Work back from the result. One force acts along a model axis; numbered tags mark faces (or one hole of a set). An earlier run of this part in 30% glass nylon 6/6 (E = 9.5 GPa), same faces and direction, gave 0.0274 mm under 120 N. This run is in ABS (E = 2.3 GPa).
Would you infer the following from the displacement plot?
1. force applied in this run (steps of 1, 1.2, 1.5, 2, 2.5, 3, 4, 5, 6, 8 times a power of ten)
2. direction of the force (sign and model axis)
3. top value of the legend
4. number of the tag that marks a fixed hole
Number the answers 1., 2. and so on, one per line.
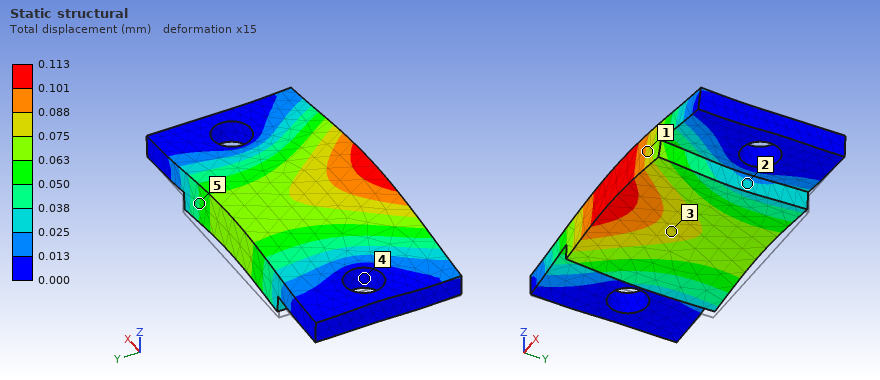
1. 120 N
2. +Z
3. 0.113 mm
4. 4
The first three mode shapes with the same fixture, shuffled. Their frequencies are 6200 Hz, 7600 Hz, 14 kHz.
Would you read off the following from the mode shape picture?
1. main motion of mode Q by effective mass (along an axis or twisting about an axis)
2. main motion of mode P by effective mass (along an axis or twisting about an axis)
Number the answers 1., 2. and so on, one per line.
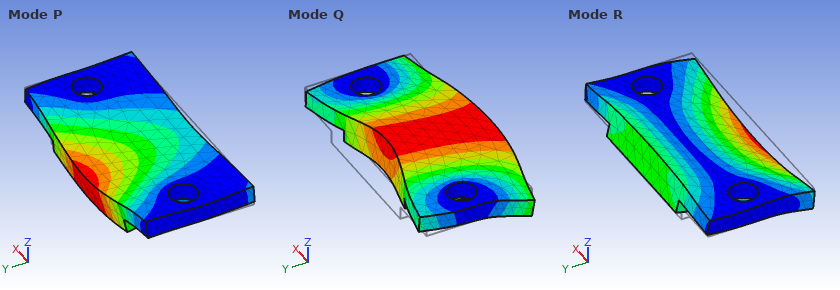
1. along Y
2. along Z
